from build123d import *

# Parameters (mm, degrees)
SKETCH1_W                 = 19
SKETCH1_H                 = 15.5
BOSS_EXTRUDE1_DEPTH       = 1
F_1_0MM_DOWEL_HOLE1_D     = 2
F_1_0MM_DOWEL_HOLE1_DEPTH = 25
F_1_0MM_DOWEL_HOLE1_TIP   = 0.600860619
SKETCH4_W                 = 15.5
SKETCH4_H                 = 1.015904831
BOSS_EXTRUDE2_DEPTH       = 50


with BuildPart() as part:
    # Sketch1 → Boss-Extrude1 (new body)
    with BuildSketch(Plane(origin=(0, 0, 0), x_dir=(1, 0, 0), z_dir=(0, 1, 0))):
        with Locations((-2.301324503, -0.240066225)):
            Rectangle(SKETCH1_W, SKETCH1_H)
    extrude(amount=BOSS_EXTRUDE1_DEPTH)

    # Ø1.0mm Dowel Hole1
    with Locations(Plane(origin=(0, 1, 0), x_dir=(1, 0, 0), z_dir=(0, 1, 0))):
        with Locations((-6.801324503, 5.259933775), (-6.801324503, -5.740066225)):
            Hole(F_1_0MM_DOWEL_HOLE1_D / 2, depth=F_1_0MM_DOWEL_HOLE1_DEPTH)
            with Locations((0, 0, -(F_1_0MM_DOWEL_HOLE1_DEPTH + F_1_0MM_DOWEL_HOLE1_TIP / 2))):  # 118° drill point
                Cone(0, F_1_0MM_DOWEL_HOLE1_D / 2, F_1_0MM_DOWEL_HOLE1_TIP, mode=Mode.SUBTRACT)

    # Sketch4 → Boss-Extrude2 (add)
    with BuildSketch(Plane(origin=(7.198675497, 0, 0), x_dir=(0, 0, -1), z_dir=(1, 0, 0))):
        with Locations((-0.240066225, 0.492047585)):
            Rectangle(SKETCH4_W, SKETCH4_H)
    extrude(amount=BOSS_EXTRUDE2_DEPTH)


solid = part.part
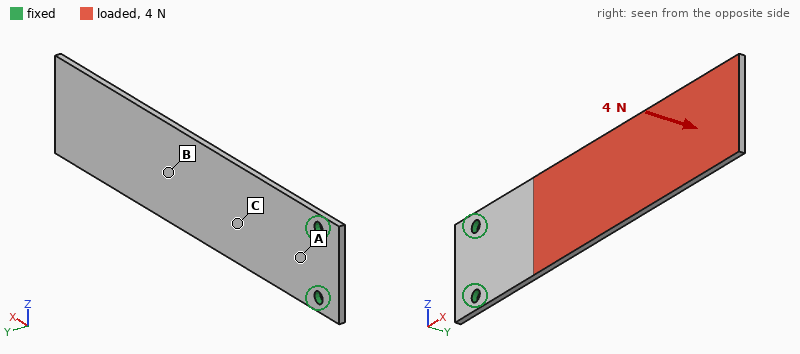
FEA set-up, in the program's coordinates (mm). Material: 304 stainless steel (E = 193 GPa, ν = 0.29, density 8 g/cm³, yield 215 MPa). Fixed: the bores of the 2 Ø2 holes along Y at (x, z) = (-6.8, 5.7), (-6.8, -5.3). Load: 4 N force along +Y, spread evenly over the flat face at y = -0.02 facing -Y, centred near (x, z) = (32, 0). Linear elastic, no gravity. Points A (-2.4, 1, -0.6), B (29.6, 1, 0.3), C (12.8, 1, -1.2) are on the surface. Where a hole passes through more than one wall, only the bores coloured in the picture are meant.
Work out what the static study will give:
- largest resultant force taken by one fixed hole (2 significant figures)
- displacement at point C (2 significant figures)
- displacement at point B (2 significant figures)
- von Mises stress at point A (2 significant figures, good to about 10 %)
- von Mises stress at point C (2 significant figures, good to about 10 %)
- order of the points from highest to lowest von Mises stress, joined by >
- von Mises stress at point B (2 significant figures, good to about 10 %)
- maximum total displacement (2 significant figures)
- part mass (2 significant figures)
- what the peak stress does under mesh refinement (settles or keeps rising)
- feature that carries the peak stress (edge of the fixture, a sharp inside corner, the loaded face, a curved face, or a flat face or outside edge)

2.0 N
0.096 mm
0.28 mm
49 MPa
29 MPa
A > C > B
12 MPa
0.63 mm
8.6 g
keeps rising
edge of the fixture
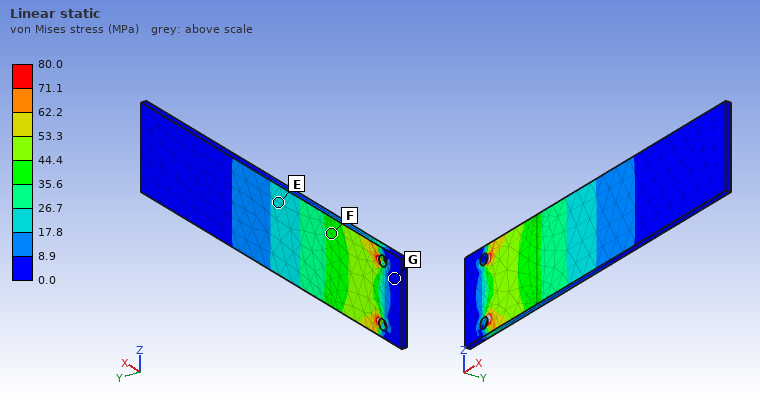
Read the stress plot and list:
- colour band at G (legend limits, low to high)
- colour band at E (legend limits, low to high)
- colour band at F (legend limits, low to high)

0.0 to 8.9 MPa
17.8 to 26.7 MPa
35.6 to 44.4 MPa
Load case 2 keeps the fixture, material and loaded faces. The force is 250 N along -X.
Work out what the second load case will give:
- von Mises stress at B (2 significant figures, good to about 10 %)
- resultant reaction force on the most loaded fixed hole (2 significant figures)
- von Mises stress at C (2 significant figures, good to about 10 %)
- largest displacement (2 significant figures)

18 MPa
130 N
28 MPa
0.80 mm
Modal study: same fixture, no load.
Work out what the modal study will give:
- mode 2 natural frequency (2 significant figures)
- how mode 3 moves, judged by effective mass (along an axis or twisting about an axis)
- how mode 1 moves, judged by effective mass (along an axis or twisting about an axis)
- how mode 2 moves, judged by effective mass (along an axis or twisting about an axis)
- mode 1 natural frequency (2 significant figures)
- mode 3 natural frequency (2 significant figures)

1200 Hz
twisting about X
along Y
along Y
200 Hz
1600 Hz
